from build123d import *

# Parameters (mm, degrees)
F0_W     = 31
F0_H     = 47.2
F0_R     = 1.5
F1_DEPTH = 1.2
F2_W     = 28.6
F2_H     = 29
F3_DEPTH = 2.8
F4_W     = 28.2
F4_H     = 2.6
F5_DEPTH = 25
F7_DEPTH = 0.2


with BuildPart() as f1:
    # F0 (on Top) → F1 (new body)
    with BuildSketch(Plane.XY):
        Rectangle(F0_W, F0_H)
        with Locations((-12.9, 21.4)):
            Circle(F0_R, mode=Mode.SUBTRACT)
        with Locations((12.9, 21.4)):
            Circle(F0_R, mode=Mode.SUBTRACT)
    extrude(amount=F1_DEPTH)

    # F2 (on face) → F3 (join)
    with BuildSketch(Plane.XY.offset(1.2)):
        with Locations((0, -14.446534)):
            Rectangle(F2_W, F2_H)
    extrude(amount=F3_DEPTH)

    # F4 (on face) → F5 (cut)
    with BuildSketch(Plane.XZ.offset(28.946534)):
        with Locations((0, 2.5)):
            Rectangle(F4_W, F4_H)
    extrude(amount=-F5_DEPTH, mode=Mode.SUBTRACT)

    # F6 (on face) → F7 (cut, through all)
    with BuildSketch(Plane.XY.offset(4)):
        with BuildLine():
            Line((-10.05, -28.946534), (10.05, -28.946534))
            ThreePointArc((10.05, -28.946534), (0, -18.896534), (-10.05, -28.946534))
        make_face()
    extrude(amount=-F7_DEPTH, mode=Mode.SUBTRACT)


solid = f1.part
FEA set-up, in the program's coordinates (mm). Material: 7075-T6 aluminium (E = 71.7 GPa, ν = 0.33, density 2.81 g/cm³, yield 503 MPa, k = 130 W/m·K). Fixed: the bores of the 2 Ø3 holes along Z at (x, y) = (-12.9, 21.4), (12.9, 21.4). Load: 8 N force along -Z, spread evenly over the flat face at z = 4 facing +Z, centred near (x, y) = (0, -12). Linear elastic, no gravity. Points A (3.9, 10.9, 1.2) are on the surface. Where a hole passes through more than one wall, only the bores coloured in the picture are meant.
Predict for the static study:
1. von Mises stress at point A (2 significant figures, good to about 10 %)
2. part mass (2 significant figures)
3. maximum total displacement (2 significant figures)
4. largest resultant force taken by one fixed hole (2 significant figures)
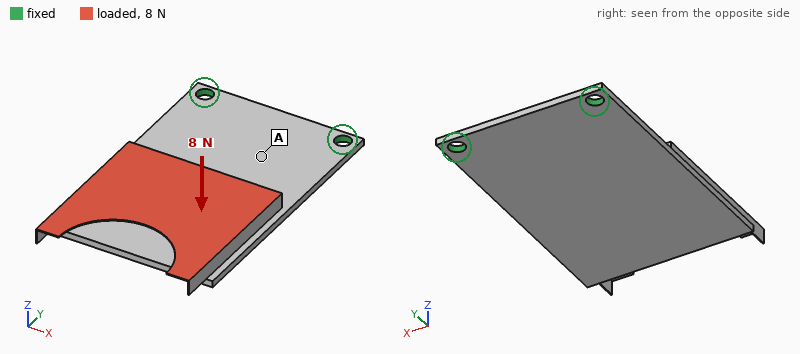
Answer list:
21 MPa
6.2 g
0.64 mm
4.0 N
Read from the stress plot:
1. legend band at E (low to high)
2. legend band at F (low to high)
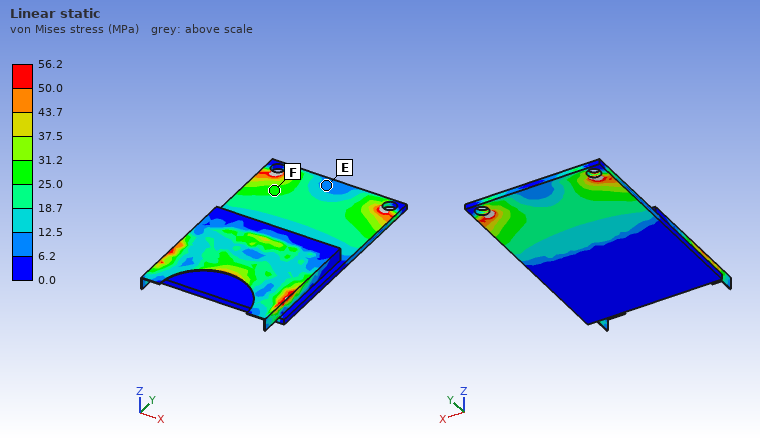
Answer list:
6.2 to 12.5 MPa
25.0 to 31.2 MPa
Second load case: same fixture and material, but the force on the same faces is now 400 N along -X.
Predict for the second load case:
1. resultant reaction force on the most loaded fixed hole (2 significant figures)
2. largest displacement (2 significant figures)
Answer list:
550 N
0.35 mm
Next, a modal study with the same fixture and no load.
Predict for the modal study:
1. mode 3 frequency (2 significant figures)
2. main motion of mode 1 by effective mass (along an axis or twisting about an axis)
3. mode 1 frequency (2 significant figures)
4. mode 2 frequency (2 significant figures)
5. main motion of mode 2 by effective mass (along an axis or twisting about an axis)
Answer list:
2200 Hz
along Z
420 Hz
1800 Hz
twisting about Y
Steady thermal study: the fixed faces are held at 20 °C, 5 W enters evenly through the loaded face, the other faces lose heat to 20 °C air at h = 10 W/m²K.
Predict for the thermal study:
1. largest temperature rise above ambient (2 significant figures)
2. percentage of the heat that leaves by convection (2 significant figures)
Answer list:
45 K
17 %
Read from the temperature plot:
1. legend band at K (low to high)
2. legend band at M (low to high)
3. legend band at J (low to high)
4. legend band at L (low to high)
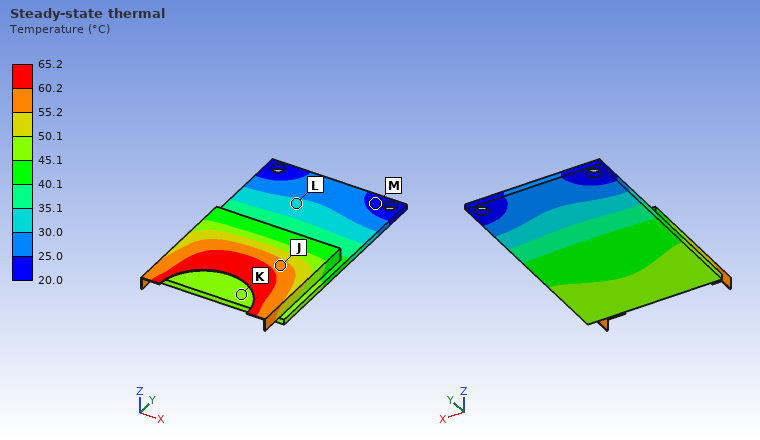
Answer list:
45.1 to 50.1 °C
20.0 to 25.0 °C
55.2 to 60.2 °C
30.0 to 35.1 °C
